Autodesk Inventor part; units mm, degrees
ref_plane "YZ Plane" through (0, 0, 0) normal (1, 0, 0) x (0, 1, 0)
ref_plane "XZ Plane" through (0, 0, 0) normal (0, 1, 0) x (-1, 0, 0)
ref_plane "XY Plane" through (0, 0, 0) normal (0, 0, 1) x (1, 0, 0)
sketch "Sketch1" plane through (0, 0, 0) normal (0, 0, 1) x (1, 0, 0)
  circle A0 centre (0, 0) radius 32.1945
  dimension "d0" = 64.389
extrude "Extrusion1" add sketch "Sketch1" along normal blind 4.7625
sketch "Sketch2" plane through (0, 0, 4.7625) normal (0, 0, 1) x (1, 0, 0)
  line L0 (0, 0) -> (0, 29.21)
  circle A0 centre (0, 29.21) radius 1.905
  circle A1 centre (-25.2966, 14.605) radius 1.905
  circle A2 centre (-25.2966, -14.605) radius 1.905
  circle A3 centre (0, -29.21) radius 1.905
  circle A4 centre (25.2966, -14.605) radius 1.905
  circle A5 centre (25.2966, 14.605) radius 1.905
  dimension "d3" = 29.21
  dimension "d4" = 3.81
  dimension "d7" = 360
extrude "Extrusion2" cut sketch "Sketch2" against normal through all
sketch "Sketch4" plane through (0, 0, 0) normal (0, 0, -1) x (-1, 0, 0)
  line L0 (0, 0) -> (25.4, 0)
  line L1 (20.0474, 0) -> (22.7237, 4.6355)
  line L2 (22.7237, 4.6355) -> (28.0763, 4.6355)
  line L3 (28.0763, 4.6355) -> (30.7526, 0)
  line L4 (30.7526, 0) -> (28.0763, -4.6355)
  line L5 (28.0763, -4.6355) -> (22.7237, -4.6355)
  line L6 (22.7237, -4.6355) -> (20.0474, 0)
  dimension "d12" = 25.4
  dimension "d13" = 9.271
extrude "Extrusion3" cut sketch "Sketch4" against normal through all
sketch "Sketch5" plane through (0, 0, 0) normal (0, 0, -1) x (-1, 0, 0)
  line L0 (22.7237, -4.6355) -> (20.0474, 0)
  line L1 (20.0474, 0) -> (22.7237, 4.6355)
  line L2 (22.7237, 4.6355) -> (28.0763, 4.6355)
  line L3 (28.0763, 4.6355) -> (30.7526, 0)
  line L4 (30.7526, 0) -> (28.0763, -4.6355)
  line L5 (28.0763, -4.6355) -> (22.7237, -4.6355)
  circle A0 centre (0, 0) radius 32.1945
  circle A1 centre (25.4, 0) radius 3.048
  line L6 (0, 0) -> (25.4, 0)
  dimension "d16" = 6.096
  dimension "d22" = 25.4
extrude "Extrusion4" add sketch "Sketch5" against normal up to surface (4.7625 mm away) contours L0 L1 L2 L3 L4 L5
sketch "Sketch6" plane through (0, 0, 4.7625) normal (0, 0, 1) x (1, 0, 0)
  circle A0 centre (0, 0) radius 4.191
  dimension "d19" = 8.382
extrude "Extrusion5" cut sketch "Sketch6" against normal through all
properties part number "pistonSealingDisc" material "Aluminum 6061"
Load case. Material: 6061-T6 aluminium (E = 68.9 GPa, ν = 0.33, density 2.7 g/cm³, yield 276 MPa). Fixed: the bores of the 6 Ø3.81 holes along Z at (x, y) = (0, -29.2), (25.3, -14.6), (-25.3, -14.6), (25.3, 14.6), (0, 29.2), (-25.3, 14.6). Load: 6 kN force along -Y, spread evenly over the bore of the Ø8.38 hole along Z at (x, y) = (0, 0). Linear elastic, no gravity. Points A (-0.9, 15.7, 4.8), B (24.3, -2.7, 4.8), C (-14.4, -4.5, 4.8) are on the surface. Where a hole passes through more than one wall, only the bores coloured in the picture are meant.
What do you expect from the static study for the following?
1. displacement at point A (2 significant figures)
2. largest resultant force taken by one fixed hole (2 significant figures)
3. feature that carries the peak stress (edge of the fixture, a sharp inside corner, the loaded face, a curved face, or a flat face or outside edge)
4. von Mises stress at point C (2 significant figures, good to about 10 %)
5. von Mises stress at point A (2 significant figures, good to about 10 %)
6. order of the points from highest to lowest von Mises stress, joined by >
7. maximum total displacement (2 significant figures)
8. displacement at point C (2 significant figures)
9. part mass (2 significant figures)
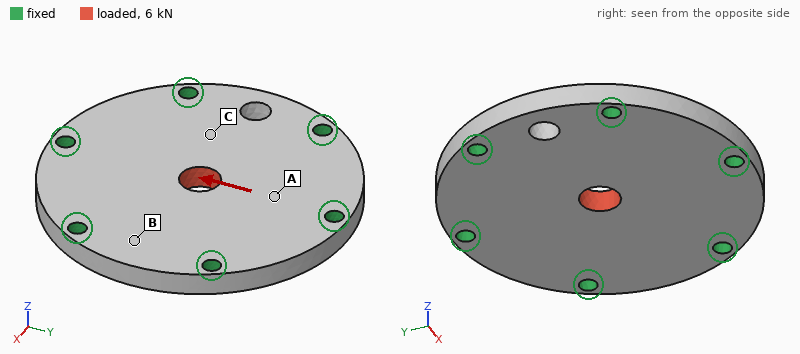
5.5 µm
1.5 kN
the loaded face
13 MPa
28 MPa
A > C > B
12 µm
3.8 µm
40 g
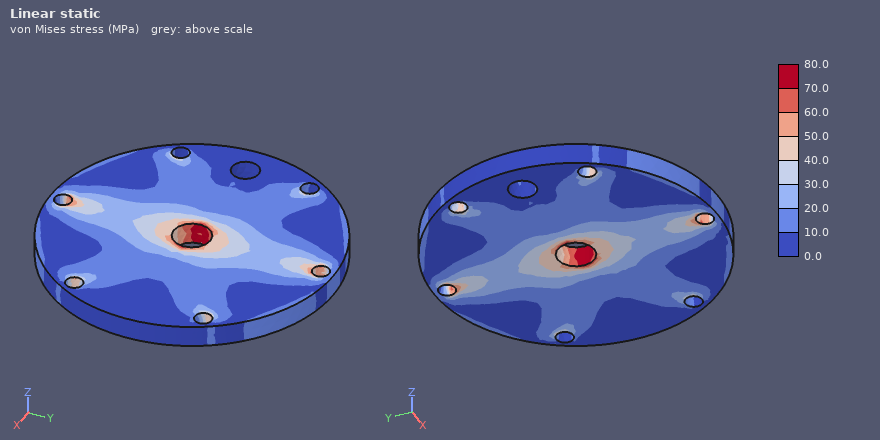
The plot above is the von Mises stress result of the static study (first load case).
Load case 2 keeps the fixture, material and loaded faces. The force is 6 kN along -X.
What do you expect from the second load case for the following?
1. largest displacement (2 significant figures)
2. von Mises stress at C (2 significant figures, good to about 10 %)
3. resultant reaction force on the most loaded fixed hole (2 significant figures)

12 µm
23 MPa
1.4 kN
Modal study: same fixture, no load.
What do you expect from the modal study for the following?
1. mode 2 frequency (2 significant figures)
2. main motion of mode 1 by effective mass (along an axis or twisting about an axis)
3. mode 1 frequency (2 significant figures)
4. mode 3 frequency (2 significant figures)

21 kHz
along Z
11 kHz
21 kHz
